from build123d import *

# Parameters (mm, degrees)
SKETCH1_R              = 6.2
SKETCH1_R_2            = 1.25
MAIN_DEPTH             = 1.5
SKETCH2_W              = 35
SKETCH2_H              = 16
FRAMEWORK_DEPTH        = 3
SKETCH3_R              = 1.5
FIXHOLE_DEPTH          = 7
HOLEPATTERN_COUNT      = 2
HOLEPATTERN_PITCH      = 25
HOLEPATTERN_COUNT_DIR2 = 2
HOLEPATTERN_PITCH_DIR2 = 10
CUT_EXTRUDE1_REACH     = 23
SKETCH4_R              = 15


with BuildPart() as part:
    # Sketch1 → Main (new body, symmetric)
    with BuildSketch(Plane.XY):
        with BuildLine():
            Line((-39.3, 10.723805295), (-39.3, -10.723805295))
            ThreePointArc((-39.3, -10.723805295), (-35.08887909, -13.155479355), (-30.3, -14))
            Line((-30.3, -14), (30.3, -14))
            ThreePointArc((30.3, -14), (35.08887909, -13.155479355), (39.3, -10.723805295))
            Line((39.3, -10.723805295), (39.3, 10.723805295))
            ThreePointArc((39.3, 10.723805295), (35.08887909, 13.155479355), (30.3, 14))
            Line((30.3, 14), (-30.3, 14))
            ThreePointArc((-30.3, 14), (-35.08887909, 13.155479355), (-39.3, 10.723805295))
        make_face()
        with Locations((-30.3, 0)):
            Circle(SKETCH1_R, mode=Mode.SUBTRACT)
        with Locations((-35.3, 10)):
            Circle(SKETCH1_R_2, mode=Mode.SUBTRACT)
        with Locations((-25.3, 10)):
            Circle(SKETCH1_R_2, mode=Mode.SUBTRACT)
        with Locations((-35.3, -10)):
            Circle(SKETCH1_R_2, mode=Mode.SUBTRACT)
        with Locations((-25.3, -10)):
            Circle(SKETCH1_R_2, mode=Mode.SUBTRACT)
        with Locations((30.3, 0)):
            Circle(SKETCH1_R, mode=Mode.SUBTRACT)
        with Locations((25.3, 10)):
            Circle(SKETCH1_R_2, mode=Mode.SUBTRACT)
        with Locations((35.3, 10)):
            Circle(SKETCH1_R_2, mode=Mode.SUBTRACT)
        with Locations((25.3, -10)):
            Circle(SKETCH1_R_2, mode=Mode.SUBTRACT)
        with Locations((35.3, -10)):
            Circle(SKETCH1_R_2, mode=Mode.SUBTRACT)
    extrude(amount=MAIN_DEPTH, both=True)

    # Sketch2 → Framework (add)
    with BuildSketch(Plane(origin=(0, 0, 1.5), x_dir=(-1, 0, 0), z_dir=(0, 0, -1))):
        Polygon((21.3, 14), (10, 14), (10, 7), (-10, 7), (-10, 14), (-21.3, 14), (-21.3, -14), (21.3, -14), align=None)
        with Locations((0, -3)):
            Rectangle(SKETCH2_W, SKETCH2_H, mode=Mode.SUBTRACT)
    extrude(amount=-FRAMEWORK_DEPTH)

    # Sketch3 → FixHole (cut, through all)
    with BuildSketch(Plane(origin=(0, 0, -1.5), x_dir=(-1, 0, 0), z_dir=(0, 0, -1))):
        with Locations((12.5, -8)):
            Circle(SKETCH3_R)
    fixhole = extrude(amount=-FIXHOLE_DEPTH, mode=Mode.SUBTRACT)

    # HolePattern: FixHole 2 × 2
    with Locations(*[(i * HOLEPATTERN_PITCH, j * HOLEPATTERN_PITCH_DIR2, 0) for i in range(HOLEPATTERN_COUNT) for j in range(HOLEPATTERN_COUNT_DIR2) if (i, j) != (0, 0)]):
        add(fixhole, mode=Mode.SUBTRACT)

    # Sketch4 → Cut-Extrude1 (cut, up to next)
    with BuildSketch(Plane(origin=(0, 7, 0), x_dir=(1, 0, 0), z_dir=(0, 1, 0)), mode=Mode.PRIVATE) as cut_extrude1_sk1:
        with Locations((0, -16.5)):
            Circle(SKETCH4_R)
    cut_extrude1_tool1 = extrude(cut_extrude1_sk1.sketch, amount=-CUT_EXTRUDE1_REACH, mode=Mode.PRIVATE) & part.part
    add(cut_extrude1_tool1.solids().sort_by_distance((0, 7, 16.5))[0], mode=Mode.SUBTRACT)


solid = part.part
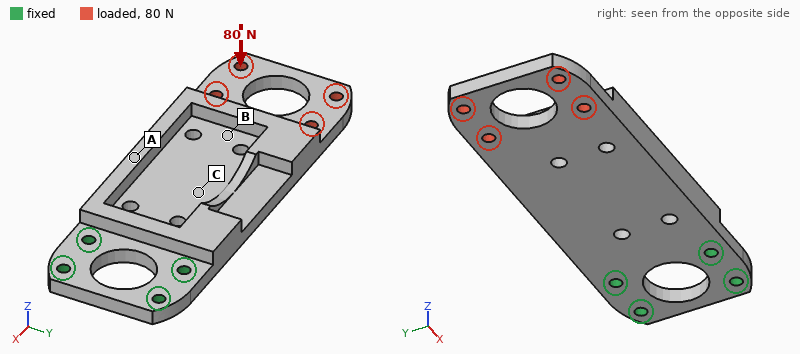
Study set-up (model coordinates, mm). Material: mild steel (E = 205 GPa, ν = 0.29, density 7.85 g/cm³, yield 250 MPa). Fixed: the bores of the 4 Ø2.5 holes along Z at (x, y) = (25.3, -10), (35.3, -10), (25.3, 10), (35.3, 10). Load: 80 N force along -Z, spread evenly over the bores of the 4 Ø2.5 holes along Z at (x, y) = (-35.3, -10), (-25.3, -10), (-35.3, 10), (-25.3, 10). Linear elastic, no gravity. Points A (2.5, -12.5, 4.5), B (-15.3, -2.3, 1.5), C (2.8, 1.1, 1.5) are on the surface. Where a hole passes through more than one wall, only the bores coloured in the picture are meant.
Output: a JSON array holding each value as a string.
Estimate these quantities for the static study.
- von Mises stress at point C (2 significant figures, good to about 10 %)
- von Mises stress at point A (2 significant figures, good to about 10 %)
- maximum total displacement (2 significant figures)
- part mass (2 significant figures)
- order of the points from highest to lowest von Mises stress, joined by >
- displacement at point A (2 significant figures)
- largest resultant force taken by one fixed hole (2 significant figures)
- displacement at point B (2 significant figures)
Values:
["32 MPa", "60 MPa", "0.27 mm", "55 g", "A > C > B", "0.061 mm", "120 N", "0.14 mm"]
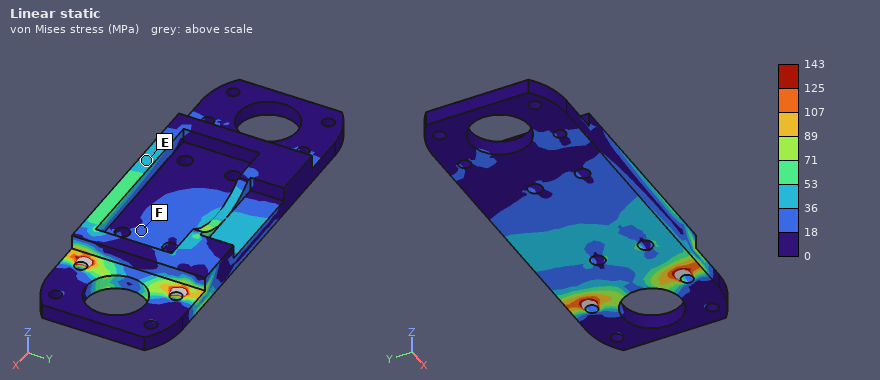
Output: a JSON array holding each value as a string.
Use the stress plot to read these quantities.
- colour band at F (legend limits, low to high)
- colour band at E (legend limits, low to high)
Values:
["18 to 36 MPa", "36 to 53 MPa"]
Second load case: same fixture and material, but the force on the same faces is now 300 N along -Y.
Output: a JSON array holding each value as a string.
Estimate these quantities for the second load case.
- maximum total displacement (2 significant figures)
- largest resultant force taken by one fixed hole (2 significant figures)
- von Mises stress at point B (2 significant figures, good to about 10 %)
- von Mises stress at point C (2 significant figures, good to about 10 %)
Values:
["26 µm", "730 N", "11 MPa", "13 MPa"]
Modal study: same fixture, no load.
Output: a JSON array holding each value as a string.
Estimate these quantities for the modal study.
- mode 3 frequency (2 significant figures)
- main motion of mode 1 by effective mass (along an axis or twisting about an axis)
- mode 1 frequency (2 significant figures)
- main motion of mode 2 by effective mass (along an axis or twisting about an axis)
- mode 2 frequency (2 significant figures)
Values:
["4500 Hz", "along Z", "780 Hz", "twisting about X", "3200 Hz"]
